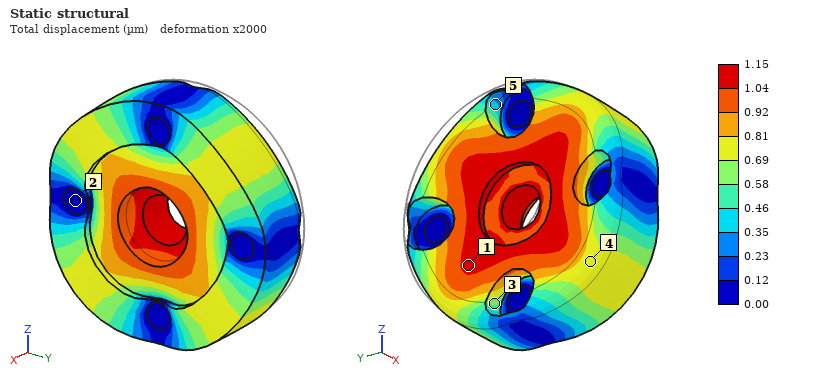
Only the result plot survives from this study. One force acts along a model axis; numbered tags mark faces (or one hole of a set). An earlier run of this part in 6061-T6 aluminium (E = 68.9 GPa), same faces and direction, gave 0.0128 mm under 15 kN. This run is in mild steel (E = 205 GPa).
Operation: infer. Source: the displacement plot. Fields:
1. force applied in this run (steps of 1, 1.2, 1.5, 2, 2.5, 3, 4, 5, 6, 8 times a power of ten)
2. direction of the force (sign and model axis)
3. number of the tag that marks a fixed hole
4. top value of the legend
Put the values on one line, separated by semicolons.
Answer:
4 kN; +X; 2; 1.15 µm
